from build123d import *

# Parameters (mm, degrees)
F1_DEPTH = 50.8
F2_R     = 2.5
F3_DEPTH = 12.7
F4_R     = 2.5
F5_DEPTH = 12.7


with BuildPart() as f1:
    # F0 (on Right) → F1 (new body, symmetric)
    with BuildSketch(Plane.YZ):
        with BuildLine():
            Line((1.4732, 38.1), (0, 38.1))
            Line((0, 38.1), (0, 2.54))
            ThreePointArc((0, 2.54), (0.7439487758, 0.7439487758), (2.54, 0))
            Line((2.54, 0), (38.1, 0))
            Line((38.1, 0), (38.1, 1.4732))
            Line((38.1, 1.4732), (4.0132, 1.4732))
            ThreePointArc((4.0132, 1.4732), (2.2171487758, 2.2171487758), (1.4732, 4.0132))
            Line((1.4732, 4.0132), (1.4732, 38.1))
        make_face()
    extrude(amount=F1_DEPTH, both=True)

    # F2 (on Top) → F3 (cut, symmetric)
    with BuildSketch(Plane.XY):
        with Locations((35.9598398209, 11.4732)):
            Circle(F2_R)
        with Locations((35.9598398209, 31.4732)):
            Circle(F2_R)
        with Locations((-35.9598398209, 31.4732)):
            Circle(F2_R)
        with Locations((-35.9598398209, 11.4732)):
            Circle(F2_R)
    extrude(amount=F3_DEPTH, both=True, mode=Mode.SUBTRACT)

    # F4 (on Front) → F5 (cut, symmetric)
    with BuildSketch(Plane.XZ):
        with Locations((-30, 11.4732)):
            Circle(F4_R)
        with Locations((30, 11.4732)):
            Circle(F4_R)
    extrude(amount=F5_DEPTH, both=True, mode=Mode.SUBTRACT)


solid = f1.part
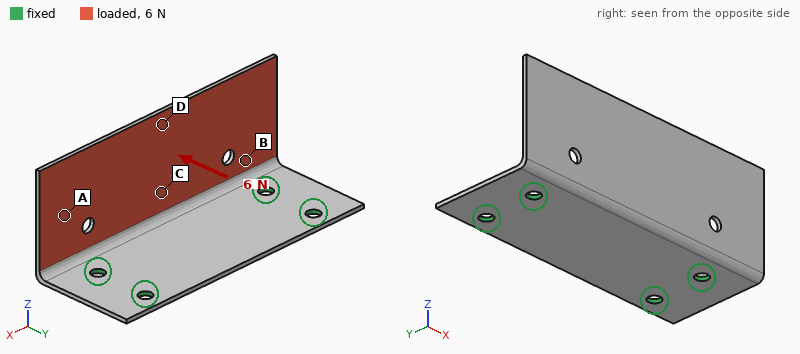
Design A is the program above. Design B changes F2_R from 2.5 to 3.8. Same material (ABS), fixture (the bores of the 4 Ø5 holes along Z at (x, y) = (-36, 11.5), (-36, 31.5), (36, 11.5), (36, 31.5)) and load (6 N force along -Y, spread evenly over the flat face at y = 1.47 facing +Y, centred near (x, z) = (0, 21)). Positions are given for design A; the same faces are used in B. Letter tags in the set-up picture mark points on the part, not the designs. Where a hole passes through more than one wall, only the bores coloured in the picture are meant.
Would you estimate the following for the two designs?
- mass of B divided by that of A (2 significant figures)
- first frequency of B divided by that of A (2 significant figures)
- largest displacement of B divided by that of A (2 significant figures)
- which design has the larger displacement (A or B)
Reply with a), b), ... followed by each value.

a) 0.99
b) 1.1
c) 0.91
d) A
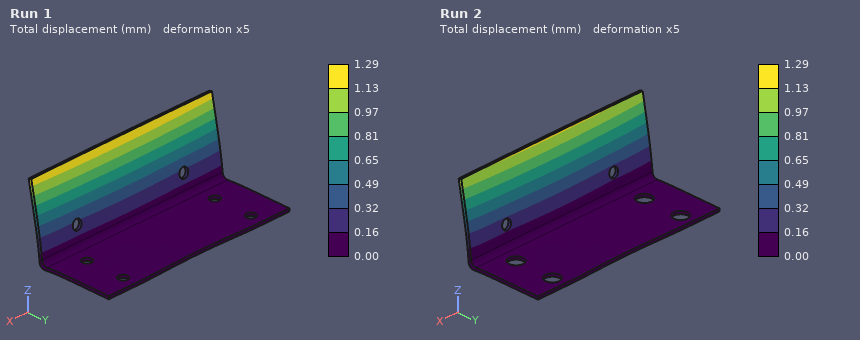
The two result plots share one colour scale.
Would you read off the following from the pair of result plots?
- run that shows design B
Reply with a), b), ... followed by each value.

a) Run 2
